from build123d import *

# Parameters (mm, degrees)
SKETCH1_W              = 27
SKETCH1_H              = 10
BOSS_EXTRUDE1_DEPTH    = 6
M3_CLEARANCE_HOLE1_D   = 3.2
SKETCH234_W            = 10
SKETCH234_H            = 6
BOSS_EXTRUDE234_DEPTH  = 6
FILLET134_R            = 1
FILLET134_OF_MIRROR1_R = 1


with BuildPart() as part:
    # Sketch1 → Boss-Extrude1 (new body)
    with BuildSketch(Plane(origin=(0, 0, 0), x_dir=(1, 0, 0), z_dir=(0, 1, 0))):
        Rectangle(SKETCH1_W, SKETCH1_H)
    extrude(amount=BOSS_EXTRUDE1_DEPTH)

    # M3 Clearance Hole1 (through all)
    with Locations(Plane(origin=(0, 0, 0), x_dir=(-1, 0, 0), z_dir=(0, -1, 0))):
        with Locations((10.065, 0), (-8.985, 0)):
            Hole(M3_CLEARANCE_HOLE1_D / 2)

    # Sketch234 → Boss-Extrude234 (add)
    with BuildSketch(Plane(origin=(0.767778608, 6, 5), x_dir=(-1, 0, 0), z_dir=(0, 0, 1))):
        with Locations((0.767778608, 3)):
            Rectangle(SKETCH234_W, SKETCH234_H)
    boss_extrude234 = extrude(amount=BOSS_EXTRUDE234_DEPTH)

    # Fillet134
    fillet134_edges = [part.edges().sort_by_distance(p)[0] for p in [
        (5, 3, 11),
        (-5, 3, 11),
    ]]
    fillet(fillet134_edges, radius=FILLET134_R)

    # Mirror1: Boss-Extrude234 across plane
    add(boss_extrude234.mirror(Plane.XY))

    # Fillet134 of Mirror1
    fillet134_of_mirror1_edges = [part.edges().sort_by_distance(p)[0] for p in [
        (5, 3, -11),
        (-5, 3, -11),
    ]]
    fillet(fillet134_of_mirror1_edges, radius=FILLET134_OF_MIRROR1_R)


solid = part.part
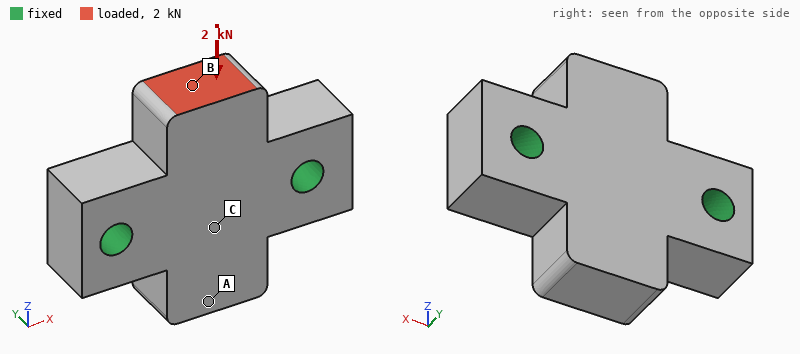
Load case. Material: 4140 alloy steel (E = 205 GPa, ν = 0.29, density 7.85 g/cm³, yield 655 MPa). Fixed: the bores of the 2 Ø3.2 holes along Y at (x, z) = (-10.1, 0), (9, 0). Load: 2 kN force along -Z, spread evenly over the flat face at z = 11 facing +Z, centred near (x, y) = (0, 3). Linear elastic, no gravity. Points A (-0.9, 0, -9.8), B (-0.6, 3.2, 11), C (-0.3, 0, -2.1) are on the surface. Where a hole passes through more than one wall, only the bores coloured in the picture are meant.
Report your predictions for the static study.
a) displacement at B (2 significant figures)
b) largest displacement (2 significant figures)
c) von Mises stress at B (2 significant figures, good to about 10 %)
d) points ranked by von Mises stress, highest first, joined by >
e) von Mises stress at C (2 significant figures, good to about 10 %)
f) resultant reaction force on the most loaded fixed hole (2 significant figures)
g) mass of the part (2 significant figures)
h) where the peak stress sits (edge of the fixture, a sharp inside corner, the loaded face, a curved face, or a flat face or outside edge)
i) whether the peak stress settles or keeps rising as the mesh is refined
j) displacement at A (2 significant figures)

3.0 µm
3.0 µm
36 MPa
B > C > A
17 MPa
1.1 kN
18 g
edge of the fixture
keeps rising
1.2 µm
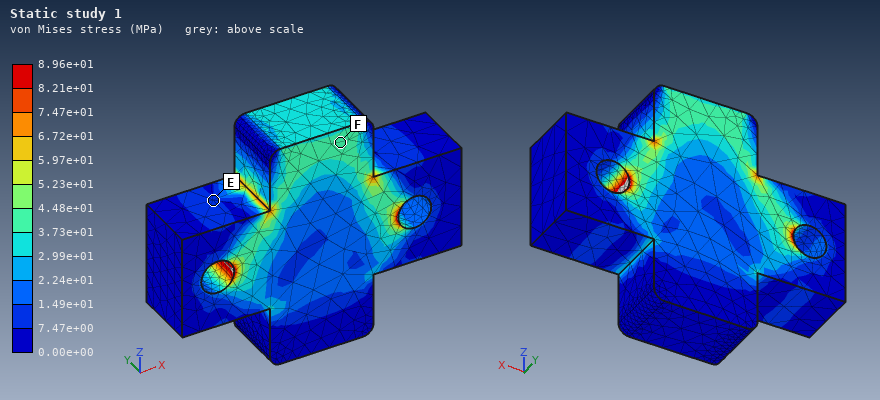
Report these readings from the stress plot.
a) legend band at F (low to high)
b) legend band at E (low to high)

3.73e+01 to 4.48e+01 MPa
7.47e+00 to 1.49e+01 MPa
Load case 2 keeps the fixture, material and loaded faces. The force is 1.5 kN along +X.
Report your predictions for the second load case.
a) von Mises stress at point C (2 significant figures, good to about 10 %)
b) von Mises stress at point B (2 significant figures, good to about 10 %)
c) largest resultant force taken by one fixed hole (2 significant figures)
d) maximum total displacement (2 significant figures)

15 MPa
55 MPa
1.2 kN
6.9 µm
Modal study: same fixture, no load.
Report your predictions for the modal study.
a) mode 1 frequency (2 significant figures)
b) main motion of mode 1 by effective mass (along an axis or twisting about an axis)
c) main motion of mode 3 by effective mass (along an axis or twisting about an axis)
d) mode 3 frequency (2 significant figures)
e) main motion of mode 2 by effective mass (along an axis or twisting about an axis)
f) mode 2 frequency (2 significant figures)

26 kHz
twisting about X
along Z
52 kHz
along Y
34 kHz
